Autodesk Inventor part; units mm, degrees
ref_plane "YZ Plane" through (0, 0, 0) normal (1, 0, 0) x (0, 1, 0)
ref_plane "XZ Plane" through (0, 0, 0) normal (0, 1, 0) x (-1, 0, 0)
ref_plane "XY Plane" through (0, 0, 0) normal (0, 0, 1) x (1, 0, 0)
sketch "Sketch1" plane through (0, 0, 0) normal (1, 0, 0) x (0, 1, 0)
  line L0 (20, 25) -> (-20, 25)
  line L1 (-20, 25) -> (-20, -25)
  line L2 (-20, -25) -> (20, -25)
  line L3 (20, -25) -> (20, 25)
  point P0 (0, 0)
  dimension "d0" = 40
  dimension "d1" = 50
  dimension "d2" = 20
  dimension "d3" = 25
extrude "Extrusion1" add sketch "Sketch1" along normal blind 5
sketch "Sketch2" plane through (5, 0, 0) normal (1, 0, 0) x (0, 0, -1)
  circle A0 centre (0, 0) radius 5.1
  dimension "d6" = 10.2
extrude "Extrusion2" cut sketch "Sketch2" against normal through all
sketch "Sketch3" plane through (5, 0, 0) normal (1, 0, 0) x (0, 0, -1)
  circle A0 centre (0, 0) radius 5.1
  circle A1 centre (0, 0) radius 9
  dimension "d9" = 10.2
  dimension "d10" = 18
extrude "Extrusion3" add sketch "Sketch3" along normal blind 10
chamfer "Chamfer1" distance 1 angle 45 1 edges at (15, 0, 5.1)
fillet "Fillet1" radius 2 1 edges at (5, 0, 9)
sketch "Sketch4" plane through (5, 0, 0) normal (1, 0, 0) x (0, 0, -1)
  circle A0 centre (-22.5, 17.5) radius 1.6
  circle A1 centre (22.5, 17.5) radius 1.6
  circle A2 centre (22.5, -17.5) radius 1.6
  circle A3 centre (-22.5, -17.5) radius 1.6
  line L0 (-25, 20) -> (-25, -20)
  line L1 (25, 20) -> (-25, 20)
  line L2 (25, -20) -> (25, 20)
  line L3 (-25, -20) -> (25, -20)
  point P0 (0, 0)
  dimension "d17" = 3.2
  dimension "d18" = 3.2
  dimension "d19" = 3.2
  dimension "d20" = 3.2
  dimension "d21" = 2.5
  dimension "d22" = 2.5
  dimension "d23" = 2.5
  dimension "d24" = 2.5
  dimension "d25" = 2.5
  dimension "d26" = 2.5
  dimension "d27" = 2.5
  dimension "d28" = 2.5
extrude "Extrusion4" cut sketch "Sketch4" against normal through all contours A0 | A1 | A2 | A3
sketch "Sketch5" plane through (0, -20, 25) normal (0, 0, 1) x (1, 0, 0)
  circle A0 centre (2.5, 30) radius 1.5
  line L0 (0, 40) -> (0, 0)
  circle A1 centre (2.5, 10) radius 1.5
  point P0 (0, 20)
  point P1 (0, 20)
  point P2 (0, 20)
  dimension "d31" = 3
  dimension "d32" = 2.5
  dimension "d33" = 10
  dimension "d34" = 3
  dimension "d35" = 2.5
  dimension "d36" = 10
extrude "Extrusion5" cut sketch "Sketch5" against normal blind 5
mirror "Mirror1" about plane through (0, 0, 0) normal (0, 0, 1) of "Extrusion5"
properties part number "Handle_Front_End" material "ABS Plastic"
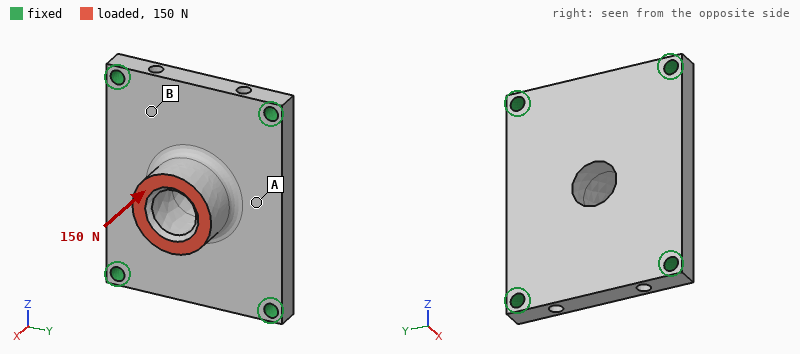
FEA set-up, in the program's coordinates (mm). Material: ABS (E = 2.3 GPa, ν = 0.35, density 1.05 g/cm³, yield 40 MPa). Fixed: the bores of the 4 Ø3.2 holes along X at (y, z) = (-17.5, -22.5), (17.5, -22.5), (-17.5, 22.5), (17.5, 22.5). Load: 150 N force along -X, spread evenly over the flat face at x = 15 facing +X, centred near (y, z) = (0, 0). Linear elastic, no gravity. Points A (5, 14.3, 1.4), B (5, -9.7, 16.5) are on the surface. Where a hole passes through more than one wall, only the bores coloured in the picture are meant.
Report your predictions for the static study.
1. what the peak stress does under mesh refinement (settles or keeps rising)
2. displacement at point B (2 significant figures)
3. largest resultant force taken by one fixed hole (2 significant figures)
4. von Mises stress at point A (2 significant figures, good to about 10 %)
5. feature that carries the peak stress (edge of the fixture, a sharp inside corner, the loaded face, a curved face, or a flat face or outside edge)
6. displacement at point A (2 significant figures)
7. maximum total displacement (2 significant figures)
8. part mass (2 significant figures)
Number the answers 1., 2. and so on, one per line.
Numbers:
1. keeps rising
2. 0.042 mm
3. 39 N
4. 2.6 MPa
5. edge of the fixture
6. 0.082 mm
7. 0.10 mm
8. 12 g
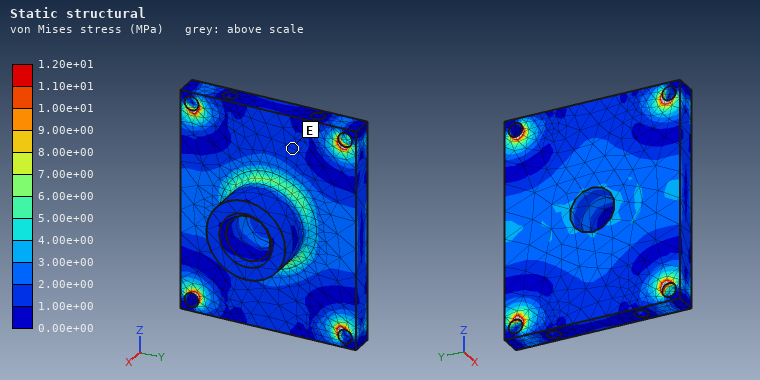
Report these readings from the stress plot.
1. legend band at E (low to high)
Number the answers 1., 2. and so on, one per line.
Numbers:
1. 1.00e+00 to 2.00e+00 MPa
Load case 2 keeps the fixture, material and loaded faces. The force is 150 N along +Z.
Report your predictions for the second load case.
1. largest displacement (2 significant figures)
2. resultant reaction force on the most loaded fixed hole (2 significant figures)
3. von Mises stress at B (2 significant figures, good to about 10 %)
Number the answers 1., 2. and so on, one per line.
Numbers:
1. 95 µm
2. 49 N
3. 1.3 MPa
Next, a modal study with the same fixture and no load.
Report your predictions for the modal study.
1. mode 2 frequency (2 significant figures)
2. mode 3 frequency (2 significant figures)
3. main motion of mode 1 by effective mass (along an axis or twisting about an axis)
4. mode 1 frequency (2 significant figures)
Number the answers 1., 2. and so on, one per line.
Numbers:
1. 3800 Hz
2. 4700 Hz
3. along X
4. 2500 Hz
